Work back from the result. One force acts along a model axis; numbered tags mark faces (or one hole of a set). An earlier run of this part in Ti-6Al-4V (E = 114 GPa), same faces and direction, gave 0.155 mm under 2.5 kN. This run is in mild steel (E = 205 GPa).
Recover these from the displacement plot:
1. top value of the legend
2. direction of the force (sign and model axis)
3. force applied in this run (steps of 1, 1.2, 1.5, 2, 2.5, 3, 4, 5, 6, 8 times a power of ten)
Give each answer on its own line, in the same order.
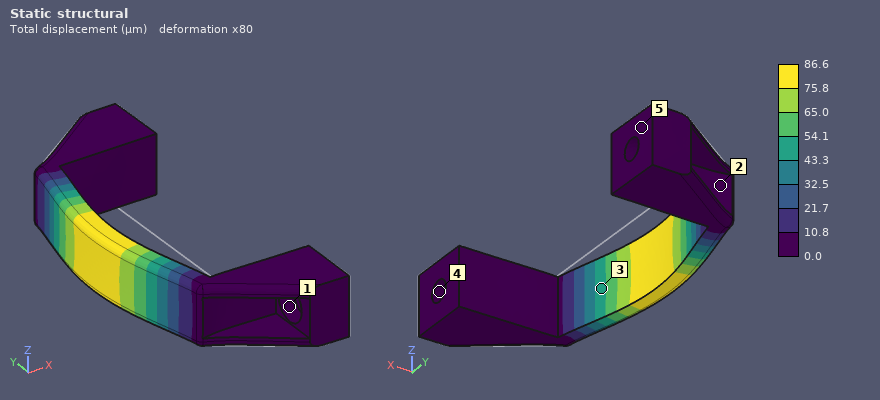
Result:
86.6 µm
-X
2.5 kN
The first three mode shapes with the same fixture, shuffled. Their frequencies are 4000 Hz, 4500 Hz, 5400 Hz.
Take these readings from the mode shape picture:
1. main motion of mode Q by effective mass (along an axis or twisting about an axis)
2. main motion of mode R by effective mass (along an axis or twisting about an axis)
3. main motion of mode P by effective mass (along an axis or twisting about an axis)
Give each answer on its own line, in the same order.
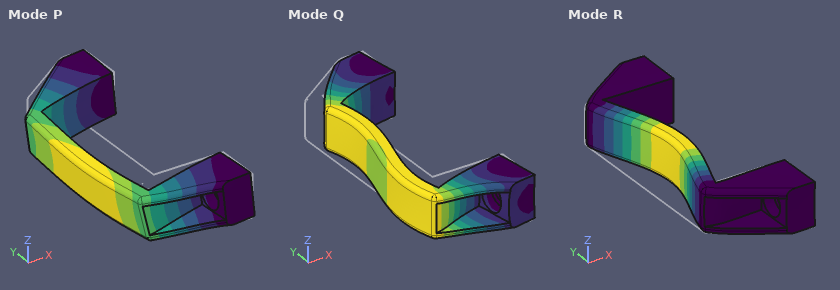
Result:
along Y
along X
along Z
